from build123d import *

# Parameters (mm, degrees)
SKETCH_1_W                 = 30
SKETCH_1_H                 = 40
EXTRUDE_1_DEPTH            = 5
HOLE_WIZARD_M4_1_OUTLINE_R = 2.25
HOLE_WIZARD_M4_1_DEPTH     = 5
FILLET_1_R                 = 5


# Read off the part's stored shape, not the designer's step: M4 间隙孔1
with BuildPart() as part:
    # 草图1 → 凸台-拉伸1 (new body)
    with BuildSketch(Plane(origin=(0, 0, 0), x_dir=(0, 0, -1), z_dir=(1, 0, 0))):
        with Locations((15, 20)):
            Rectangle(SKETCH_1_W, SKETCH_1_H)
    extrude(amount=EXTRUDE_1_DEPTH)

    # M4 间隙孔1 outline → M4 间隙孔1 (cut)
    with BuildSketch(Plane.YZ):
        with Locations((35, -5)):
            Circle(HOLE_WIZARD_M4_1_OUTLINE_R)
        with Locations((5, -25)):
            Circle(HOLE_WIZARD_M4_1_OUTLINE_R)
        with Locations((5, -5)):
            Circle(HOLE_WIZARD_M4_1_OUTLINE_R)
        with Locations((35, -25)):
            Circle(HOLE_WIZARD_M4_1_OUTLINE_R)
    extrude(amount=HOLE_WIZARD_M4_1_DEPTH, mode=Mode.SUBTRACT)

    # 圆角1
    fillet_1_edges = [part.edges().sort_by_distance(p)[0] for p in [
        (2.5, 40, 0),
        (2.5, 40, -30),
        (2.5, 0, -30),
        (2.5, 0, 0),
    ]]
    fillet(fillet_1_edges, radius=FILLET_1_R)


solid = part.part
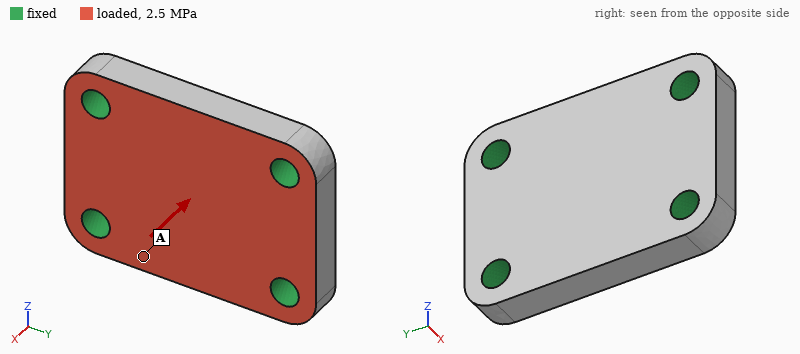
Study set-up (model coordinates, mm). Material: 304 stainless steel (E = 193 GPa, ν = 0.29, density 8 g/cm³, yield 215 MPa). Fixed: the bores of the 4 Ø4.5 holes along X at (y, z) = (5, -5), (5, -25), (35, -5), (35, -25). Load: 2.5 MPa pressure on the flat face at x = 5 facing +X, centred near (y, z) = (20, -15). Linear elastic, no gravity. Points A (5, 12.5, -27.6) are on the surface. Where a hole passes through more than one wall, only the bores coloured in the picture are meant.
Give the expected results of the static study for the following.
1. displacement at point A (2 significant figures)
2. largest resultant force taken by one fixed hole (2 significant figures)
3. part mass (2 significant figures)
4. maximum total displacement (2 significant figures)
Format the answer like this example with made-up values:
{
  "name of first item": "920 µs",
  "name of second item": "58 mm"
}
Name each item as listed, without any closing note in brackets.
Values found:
{
  "displacement at point A": "1.8 µm",
  "largest resultant force taken by one fixed hole": "700 N",
  "part mass": "45 g",
  "maximum total displacement": "3.4 µm"
}
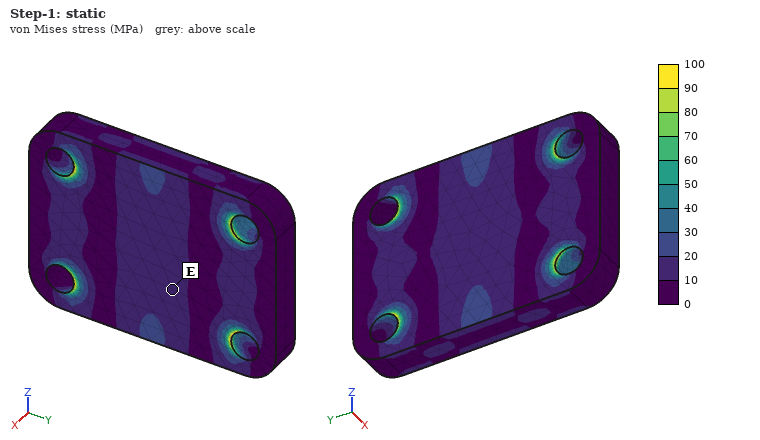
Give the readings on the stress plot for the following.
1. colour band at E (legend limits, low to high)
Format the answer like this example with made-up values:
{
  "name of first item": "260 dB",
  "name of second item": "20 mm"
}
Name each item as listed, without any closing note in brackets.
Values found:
{
  "colour band at E": "10 to 20 MPa"
}
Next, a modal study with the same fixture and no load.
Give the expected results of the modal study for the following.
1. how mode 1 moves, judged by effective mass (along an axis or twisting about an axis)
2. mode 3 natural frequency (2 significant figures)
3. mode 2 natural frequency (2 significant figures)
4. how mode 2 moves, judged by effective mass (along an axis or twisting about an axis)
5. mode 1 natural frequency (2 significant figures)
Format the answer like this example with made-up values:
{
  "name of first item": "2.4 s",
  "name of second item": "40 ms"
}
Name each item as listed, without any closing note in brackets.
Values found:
{
  "how mode 1 moves, judged by effective mass": "along X",
  "mode 3 natural frequency": "43 kHz",
  "mode 2 natural frequency": "31 kHz",
  "how mode 2 moves, judged by effective mass": "twisting about Y",
  "mode 1 natural frequency": "25 kHz"
}
